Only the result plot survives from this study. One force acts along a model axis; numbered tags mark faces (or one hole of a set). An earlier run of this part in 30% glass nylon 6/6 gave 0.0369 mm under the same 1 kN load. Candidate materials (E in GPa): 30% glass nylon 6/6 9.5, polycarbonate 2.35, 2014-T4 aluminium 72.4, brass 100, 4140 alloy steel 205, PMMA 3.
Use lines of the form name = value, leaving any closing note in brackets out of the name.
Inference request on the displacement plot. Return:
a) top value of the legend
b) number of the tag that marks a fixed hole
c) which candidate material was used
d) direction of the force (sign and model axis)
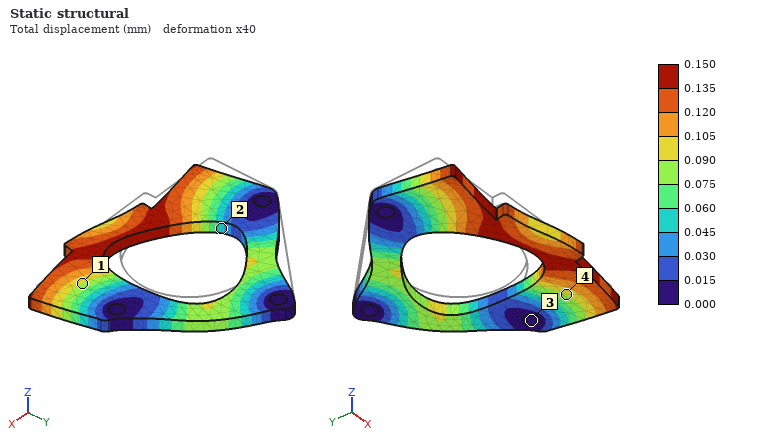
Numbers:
top value of the legend = 0.150 mm
number of the tag that marks a fixed hole = 3
which candidate material was used = polycarbonate
direction of the force = +X
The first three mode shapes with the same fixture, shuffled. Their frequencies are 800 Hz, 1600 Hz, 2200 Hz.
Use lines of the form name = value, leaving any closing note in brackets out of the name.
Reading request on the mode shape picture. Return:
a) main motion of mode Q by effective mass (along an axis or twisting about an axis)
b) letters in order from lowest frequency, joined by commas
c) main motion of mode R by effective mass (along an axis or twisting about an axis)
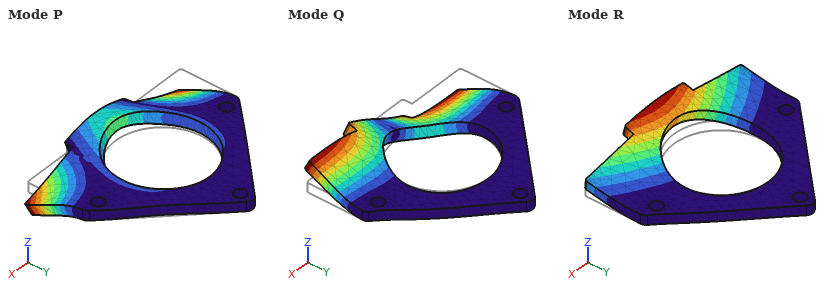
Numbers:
main motion of mode Q by effective mass = twisting about Y
letters in order from lowest frequency, joined by commas = R, Q, P
main motion of mode R by effective mass = along Z
